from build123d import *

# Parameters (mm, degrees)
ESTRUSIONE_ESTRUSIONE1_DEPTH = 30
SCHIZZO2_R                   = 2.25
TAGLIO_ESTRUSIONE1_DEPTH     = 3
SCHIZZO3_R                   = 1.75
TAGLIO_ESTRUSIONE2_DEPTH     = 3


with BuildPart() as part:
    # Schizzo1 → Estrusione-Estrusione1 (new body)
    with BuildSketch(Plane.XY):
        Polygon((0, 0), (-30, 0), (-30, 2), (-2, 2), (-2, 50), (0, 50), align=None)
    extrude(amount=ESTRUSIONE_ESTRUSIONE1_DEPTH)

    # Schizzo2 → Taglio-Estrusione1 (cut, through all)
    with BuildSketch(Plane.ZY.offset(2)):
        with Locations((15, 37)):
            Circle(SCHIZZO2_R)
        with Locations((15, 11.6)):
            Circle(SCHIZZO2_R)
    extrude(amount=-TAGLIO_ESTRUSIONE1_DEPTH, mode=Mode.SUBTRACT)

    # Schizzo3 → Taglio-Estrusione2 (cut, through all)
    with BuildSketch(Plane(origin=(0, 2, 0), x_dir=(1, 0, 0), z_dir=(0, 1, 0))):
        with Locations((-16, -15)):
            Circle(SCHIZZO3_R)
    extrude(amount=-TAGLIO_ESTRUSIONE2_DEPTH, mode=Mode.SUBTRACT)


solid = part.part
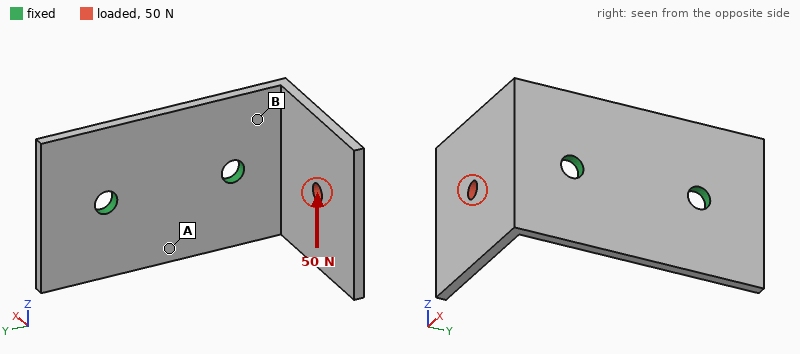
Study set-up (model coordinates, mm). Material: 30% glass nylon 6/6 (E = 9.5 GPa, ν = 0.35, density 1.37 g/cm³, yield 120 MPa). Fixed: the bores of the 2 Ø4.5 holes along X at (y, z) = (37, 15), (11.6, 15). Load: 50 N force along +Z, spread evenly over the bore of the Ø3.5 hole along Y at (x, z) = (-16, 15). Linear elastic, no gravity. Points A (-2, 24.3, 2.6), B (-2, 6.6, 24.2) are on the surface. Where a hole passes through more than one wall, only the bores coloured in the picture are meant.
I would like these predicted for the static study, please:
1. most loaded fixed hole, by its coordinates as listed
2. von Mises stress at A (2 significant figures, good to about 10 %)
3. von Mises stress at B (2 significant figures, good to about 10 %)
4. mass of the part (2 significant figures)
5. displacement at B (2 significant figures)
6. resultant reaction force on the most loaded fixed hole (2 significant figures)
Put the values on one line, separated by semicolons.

(11.6, 15); 4.8 MPa; 11 MPa; 6.3 g; 0.12 mm; 66 N
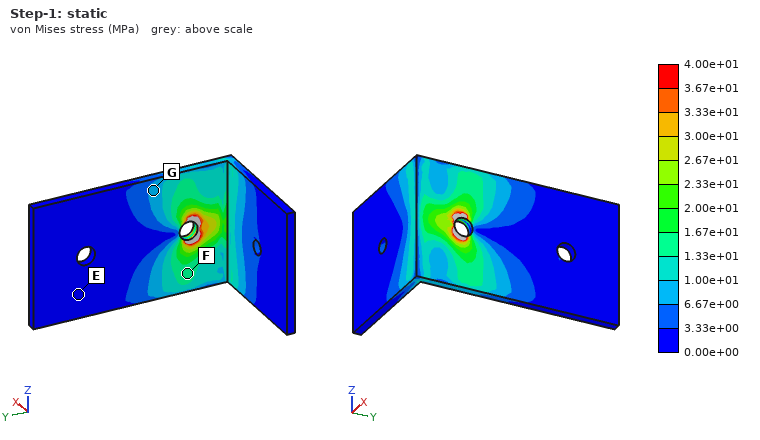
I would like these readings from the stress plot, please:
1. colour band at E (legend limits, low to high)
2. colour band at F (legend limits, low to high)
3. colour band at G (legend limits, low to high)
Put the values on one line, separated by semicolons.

0.00e+00 to 3.33e+00 MPa; 1.33e+01 to 1.67e+01 MPa; 6.67e+00 to 1.00e+01 MPa
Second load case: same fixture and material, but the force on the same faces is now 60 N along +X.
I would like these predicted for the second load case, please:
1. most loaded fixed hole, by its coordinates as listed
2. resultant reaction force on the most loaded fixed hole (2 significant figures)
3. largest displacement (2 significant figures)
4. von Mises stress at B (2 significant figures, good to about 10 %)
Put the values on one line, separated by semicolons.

(11.6, 15); 65 N; 0.51 mm; 12 MPa
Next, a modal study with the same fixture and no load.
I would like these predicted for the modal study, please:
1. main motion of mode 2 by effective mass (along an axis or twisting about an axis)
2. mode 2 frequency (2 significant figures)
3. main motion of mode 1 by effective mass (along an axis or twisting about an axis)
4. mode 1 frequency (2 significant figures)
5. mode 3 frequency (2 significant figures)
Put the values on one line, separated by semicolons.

along Z; 1000 Hz; along Y; 660 Hz; 2200 Hz
